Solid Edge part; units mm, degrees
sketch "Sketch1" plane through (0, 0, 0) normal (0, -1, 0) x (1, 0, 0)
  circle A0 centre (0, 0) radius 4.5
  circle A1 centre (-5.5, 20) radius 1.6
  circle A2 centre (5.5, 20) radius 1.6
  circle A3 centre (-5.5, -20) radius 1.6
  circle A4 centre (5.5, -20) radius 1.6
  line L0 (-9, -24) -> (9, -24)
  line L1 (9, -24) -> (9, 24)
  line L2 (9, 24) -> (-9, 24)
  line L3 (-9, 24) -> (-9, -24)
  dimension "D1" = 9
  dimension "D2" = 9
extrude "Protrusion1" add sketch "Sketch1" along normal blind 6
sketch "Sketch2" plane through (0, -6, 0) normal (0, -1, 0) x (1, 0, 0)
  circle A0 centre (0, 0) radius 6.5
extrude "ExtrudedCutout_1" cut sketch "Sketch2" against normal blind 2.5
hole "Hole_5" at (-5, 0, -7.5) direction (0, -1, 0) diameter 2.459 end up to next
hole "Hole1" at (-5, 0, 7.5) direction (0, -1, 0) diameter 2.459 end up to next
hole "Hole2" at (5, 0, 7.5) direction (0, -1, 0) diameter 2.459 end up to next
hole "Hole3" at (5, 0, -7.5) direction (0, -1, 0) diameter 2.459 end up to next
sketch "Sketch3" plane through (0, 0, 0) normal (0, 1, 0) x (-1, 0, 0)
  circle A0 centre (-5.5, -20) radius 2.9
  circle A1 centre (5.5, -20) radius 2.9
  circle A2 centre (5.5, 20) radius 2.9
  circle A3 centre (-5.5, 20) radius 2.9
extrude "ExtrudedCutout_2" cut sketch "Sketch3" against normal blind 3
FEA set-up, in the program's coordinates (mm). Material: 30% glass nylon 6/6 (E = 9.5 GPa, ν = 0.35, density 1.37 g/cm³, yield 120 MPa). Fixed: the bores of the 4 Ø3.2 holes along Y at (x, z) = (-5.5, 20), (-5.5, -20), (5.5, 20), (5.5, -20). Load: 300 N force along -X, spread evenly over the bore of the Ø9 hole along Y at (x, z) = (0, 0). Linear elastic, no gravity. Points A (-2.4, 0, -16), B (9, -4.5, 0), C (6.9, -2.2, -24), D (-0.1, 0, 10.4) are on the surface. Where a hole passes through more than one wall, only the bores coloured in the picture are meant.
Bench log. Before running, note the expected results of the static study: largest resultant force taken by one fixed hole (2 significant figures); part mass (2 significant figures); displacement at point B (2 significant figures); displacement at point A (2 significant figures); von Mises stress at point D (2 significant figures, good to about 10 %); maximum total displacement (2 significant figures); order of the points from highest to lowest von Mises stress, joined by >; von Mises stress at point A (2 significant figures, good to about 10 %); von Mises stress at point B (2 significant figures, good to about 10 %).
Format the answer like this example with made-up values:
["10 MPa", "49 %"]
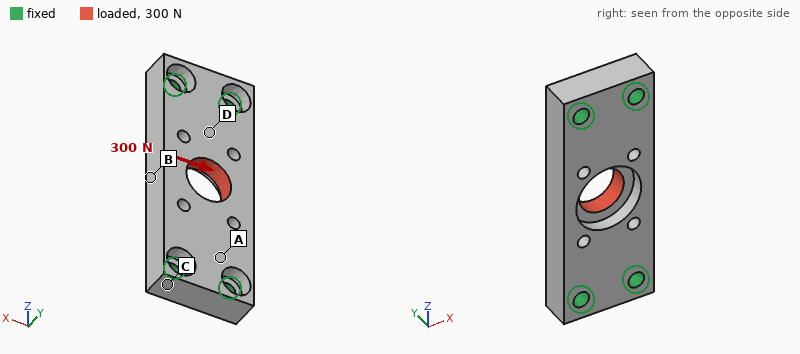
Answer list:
["130 N", "5.6 g", "14 µm", "4.0 µm", "4.4 MPa", "18 µm", "B > D > A > C", "2.5 MPa", "6.1 MPa"]
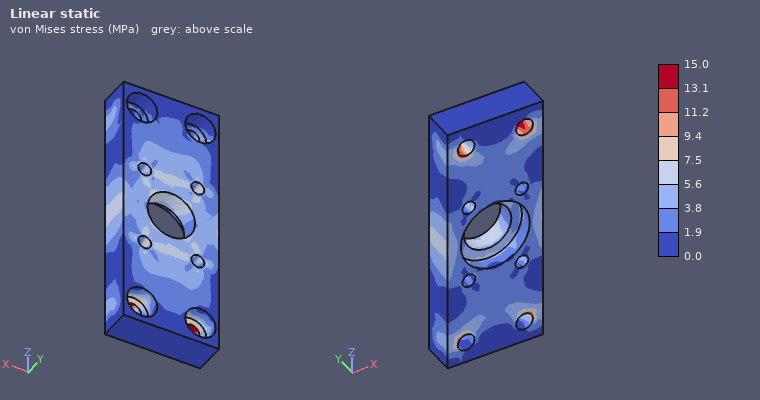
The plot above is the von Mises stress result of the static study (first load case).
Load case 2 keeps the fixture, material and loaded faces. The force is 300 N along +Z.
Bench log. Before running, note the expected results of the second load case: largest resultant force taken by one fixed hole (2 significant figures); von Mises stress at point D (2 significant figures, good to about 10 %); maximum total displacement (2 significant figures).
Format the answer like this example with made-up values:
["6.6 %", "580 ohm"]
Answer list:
["76 N", "2.3 MPa", "5.4 µm"]
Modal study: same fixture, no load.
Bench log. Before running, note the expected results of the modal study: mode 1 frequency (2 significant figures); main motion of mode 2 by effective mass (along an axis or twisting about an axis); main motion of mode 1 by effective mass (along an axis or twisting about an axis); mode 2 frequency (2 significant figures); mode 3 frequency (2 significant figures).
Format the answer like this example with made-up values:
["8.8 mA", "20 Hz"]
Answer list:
["7500 Hz", "twisting about Z", "along Y", "12 kHz", "16 kHz"]
